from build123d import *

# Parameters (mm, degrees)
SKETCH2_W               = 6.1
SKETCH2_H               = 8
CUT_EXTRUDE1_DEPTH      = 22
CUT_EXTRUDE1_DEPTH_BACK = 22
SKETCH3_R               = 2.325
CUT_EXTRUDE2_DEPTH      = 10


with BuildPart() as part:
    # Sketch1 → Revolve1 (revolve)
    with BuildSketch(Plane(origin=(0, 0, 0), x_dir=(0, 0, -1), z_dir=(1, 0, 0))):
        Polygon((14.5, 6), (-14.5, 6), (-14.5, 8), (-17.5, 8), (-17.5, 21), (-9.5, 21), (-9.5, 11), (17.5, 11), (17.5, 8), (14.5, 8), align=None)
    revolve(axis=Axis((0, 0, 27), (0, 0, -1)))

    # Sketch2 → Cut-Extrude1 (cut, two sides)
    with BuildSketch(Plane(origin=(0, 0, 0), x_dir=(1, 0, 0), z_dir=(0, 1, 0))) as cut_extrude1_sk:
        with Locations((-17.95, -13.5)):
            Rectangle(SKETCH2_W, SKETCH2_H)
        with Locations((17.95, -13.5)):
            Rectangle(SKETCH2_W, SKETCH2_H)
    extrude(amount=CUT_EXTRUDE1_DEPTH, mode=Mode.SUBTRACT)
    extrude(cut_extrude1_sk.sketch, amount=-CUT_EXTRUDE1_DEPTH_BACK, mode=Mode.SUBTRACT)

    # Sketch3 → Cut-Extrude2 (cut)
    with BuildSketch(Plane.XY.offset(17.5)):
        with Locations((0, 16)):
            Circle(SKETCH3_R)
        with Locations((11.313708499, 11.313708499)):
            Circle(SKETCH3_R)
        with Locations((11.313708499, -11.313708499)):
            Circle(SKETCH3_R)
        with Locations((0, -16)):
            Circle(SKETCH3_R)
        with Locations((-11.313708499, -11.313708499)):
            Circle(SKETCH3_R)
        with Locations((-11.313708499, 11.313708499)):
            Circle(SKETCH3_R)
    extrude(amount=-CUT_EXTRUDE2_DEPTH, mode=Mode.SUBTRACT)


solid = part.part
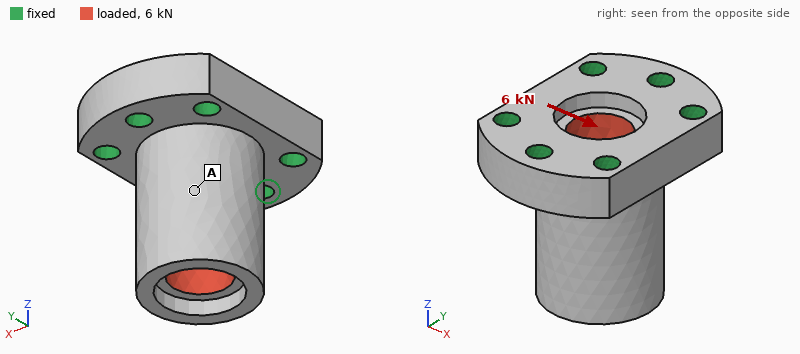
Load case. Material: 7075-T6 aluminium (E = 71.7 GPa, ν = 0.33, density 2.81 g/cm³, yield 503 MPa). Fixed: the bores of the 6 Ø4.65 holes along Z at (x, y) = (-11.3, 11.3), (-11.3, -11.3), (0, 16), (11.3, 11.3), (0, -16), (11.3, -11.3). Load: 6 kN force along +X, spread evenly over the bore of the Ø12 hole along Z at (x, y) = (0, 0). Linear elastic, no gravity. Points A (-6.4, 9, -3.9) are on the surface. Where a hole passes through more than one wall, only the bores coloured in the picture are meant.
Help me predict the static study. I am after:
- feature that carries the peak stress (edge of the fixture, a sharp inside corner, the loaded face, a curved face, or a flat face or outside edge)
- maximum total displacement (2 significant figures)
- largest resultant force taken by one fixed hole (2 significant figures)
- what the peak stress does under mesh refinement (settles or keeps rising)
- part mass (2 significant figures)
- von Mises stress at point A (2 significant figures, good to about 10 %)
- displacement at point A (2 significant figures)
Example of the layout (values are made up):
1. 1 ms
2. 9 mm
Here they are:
1. edge of the fixture
2. 51 µm
3. 2.3 kN
4. keeps rising
5. 39 g
6. 19 MPa
7. 29 µm
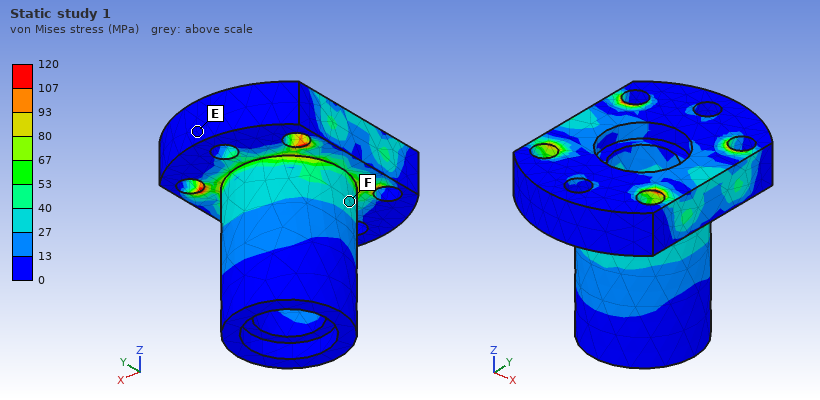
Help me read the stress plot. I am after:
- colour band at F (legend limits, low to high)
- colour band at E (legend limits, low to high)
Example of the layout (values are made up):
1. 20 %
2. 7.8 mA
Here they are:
1. 27 to 40 MPa
2. 0 to 13 MPa
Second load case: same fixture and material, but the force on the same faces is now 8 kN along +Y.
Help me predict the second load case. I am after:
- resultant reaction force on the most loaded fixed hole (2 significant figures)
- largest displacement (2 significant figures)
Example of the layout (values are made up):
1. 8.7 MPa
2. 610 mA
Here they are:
1. 2.6 kN
2. 56 µm
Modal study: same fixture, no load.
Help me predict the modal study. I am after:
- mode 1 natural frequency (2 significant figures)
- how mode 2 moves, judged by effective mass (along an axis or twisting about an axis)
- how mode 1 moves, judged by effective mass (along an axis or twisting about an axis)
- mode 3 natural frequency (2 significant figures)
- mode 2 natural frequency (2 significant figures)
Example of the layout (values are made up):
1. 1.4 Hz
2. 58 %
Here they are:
1. 13 kHz
2. along Y
3. along X
4. 26 kHz
5. 14 kHz
